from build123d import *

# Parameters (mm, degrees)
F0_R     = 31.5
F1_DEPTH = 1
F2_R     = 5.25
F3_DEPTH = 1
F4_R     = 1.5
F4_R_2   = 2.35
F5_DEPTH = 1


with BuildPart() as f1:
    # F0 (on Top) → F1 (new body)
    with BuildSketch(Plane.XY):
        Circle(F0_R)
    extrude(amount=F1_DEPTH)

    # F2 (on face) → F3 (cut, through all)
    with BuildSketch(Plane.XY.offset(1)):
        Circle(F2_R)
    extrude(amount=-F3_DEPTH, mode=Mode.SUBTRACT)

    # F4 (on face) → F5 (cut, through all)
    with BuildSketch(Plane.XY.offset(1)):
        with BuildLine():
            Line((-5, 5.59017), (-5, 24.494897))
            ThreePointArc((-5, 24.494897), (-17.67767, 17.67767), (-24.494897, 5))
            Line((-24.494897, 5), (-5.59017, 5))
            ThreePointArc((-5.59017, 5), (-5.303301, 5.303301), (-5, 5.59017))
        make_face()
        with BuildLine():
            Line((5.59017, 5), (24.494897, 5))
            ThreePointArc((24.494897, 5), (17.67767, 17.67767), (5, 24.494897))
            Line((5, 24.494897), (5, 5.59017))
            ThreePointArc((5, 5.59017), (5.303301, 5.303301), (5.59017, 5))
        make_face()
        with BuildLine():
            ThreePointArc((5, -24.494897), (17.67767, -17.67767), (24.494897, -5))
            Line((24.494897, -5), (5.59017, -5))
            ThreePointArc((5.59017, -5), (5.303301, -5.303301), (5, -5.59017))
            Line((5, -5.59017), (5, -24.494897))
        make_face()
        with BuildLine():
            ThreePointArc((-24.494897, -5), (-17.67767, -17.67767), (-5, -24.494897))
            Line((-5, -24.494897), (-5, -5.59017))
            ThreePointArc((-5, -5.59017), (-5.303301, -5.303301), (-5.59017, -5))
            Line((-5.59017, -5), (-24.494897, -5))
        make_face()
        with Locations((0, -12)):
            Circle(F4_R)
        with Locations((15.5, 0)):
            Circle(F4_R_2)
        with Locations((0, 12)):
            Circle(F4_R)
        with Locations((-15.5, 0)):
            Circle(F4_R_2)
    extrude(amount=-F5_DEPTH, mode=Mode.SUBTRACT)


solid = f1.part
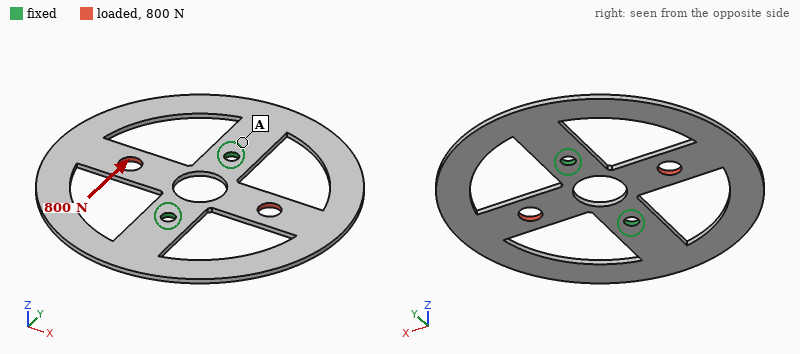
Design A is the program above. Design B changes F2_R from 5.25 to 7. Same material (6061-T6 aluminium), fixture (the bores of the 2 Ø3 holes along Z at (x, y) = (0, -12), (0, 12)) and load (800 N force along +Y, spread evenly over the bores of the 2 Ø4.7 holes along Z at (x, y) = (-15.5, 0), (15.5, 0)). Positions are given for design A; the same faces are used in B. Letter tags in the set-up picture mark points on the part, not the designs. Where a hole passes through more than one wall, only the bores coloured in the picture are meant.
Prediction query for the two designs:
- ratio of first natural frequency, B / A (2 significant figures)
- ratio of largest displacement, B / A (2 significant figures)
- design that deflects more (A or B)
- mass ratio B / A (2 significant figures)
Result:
0.82
1.3
B
0.96
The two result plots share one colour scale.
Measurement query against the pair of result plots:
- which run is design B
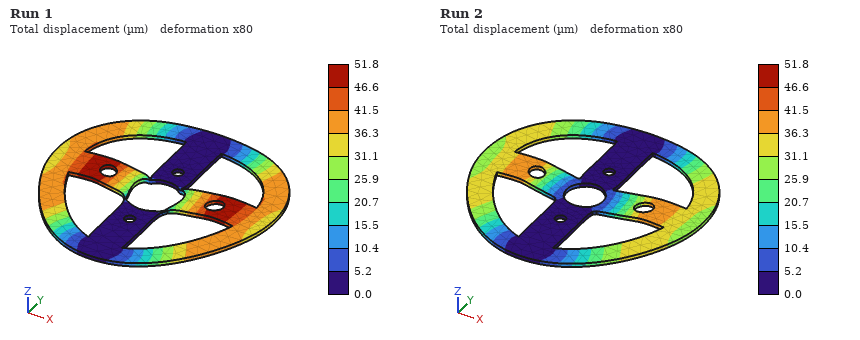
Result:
Run 1
